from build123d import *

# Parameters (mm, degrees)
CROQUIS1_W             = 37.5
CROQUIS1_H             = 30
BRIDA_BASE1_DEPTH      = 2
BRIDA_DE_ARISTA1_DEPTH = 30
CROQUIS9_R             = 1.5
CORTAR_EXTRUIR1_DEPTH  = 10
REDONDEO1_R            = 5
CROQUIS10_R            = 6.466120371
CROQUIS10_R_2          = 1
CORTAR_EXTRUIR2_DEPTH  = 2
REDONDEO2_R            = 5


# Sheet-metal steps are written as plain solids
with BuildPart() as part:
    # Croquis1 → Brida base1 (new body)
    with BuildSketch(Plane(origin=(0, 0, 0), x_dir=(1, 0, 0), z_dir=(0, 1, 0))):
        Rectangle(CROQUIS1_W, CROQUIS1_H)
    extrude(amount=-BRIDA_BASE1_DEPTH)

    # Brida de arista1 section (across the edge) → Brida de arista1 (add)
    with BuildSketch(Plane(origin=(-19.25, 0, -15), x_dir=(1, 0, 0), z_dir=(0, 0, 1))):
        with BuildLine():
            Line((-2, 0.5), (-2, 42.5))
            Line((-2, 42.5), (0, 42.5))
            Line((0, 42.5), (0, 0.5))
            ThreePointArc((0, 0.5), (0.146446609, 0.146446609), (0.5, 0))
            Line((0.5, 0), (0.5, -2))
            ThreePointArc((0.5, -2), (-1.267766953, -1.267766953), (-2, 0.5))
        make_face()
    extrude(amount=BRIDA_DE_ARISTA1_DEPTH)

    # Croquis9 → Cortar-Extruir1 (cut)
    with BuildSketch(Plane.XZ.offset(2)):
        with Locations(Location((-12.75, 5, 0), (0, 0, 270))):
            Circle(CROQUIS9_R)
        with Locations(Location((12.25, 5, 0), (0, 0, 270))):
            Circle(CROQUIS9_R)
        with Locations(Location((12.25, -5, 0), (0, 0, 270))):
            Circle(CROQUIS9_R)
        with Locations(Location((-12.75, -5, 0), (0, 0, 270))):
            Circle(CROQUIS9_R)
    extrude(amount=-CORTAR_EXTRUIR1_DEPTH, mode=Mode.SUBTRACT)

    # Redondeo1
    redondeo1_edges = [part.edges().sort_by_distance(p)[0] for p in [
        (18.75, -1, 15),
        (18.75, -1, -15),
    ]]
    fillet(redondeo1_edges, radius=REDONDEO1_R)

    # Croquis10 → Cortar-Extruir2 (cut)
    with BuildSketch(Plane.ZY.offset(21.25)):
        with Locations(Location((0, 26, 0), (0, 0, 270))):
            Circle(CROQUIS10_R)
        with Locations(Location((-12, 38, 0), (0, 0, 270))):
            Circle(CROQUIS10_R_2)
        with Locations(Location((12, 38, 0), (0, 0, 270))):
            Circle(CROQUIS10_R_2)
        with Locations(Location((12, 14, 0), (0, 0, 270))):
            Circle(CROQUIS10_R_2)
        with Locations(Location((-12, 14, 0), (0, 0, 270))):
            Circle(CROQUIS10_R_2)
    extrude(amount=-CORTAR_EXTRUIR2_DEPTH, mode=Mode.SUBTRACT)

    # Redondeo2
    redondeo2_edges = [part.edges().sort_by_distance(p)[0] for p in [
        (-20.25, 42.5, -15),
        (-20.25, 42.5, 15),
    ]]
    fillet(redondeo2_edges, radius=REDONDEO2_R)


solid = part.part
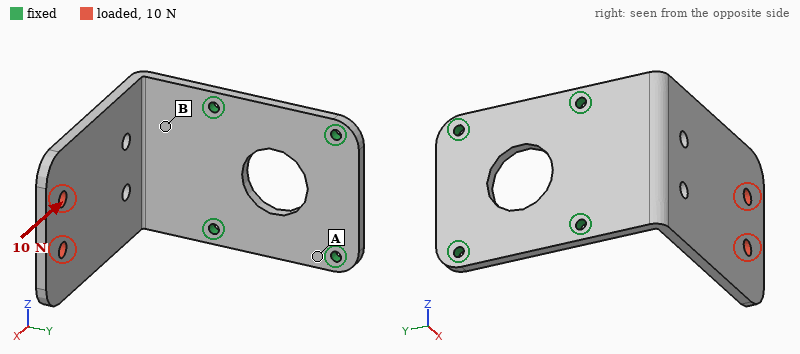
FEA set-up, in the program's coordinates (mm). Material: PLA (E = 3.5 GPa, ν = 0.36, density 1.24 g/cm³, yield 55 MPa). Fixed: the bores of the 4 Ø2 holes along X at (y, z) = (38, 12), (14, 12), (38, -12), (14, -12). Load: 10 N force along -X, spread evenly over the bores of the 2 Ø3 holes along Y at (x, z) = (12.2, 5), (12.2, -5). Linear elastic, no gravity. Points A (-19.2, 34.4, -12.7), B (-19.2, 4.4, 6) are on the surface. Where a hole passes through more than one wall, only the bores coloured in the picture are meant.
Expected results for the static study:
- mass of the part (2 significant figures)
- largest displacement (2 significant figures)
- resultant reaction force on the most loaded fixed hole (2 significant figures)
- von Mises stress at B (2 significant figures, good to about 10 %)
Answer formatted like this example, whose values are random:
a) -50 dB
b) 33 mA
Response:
a) 5.6 g
b) 0.72 mm
c) 5.8 N
d) 2.5 MPa
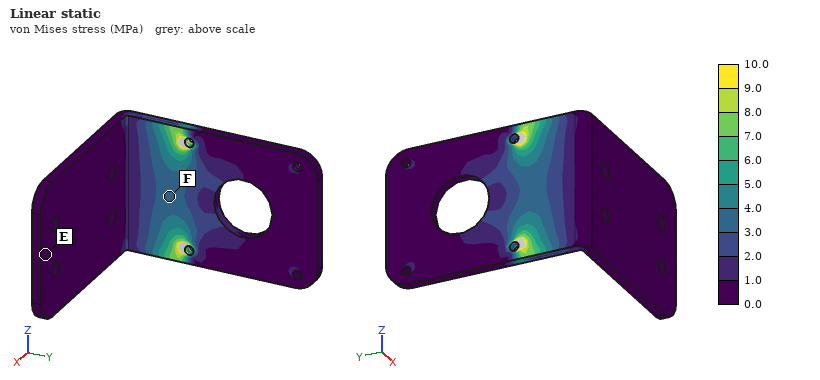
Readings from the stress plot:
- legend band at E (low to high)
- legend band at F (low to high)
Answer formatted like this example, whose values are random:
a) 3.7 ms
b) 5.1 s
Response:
a) 0.0 to 1.0 MPa
b) 3.0 to 4.0 MPa
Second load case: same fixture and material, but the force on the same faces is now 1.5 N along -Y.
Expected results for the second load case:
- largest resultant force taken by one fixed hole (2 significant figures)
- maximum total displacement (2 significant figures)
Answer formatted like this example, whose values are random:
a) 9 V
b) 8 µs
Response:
a) 0.78 N
b) 0.72 mm
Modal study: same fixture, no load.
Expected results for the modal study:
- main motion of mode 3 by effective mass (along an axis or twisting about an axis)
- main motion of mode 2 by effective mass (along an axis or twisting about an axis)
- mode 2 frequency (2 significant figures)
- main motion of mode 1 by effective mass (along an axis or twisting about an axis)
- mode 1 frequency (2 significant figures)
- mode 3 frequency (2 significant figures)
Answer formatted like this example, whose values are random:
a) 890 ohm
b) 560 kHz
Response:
a) along X
b) along Z
c) 510 Hz
d) along Y
e) 230 Hz
f) 880 Hz
